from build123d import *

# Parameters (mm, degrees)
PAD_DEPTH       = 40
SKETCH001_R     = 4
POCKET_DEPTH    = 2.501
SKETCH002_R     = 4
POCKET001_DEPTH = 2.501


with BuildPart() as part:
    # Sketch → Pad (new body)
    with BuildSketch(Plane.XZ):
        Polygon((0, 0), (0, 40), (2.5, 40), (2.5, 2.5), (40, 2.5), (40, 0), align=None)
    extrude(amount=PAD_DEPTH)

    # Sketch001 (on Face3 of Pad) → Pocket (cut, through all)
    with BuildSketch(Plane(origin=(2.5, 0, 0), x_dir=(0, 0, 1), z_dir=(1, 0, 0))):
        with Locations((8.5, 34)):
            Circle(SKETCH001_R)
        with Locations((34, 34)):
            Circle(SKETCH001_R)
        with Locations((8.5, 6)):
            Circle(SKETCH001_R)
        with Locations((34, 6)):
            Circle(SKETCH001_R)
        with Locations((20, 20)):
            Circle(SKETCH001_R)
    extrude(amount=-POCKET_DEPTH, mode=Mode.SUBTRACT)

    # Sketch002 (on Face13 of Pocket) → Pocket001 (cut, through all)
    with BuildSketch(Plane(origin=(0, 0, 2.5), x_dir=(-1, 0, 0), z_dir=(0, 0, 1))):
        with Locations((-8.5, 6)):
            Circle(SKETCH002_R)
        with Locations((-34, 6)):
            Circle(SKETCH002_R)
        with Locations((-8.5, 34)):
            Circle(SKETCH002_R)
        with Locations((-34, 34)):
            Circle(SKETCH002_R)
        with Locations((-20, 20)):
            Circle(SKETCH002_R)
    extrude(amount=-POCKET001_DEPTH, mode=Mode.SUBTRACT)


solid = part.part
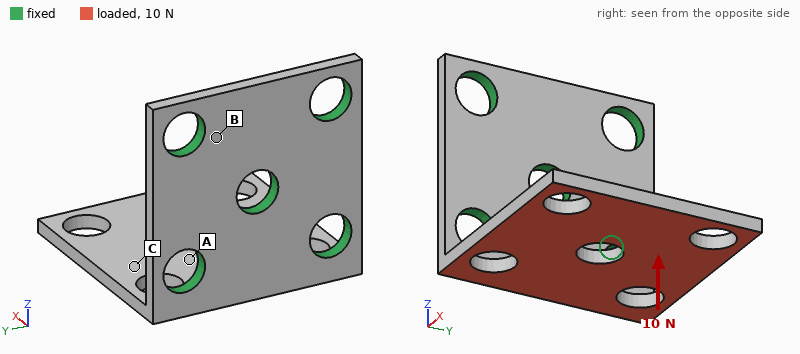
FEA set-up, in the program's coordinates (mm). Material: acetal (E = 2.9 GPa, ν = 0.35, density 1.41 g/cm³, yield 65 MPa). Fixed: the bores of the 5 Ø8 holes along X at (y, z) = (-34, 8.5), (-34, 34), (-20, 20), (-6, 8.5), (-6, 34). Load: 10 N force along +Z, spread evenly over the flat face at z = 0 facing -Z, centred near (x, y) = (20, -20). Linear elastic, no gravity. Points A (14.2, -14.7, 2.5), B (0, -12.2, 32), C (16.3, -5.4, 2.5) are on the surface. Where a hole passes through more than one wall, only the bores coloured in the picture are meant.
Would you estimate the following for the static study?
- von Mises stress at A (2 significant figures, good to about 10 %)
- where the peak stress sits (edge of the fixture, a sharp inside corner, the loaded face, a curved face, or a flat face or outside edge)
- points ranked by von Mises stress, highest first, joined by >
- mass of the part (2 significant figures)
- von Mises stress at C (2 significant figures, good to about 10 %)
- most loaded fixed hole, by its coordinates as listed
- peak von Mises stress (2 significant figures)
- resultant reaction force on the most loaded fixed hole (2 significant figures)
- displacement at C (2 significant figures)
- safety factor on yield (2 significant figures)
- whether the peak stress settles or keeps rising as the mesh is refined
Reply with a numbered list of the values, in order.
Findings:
1. 2.7 MPa
2. the loaded face
3. A > C > B
4. 9.2 g
5. 1.3 MPa
6. (-20, 20)
7. 8.7 MPa
8. 5.4 N
9. 0.20 mm
10. 7.4
11. settles
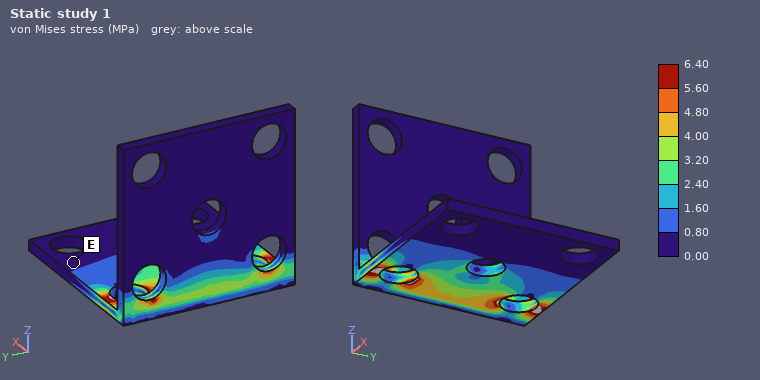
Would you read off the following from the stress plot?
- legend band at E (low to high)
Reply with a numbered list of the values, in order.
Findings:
1. 0.00 to 0.80 MPa
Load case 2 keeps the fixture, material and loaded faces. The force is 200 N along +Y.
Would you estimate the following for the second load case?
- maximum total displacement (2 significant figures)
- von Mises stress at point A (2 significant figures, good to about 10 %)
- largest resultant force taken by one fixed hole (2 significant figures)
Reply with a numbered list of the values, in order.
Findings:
1. 0.38 mm
2. 2.1 MPa
3. 160 N
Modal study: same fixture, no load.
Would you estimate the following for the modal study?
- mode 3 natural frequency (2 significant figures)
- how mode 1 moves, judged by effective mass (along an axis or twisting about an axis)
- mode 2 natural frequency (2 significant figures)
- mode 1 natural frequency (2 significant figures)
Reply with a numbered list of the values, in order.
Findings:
1. 2000 Hz
2. along Z
3. 840 Hz
4. 330 Hz
